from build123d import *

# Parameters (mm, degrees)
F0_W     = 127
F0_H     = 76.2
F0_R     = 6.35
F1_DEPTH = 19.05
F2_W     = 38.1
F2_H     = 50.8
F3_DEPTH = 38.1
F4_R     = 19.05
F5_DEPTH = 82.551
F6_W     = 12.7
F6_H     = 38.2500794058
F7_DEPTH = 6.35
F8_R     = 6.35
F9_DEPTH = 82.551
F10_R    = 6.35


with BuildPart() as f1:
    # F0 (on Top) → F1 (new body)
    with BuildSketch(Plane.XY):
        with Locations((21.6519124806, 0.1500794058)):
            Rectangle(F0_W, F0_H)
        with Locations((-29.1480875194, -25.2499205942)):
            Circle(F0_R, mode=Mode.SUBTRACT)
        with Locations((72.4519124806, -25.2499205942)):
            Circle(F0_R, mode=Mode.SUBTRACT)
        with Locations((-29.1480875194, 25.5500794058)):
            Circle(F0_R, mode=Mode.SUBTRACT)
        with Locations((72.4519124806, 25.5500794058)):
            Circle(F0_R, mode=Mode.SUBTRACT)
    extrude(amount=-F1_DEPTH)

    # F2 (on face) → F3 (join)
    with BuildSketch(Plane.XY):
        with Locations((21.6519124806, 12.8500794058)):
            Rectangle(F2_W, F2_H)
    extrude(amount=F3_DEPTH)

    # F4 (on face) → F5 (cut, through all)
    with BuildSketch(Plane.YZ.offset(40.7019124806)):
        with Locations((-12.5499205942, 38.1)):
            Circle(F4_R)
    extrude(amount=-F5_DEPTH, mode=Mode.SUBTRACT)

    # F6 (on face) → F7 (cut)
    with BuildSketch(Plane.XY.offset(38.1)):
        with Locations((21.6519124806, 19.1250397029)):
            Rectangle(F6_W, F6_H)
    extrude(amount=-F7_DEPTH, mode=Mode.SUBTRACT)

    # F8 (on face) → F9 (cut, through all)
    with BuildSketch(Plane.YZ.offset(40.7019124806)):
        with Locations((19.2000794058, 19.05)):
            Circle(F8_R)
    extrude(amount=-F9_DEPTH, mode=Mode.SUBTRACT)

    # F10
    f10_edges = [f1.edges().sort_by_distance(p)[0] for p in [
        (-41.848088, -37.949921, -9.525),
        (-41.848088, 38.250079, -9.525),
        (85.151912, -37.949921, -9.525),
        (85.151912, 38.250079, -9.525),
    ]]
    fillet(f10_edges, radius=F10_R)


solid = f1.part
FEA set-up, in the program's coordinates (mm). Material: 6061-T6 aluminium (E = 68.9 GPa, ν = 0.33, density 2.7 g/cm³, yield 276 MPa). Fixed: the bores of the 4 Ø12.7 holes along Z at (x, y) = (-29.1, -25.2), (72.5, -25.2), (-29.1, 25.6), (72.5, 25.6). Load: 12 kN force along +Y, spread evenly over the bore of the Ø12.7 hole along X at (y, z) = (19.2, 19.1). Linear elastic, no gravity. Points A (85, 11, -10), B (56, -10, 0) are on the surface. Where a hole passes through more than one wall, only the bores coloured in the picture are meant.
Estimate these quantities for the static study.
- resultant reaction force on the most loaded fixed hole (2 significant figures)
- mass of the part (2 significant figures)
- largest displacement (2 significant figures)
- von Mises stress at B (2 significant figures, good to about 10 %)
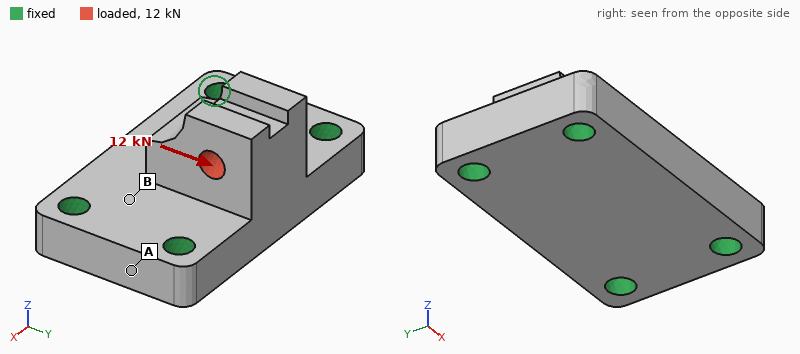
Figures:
5.1 kN
620 g
64 µm
21 MPa
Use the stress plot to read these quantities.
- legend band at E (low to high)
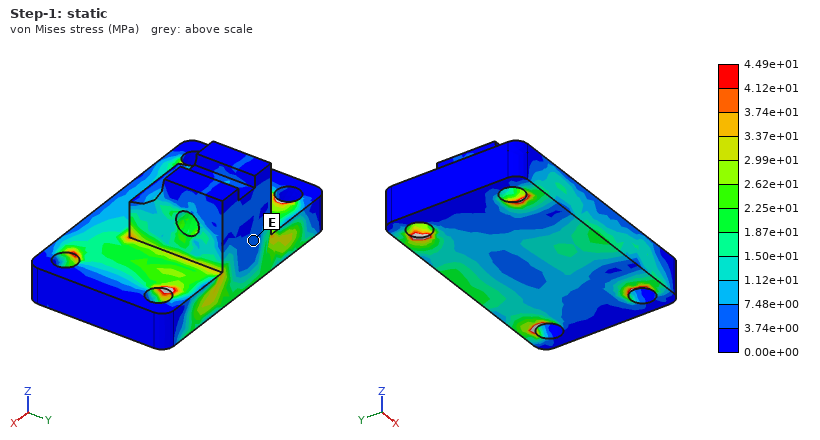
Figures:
3.74e+00 to 7.48e+00 MPa
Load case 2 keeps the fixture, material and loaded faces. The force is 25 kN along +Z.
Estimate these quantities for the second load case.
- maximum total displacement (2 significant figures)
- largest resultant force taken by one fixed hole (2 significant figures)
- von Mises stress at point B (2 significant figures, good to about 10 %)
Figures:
80 µm
11 kN
15 MPa
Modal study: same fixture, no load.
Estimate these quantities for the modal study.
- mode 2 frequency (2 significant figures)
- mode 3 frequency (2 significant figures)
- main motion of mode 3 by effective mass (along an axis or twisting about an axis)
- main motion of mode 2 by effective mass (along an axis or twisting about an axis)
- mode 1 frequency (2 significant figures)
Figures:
7200 Hz
8900 Hz
along X
along Z
6000 Hz
